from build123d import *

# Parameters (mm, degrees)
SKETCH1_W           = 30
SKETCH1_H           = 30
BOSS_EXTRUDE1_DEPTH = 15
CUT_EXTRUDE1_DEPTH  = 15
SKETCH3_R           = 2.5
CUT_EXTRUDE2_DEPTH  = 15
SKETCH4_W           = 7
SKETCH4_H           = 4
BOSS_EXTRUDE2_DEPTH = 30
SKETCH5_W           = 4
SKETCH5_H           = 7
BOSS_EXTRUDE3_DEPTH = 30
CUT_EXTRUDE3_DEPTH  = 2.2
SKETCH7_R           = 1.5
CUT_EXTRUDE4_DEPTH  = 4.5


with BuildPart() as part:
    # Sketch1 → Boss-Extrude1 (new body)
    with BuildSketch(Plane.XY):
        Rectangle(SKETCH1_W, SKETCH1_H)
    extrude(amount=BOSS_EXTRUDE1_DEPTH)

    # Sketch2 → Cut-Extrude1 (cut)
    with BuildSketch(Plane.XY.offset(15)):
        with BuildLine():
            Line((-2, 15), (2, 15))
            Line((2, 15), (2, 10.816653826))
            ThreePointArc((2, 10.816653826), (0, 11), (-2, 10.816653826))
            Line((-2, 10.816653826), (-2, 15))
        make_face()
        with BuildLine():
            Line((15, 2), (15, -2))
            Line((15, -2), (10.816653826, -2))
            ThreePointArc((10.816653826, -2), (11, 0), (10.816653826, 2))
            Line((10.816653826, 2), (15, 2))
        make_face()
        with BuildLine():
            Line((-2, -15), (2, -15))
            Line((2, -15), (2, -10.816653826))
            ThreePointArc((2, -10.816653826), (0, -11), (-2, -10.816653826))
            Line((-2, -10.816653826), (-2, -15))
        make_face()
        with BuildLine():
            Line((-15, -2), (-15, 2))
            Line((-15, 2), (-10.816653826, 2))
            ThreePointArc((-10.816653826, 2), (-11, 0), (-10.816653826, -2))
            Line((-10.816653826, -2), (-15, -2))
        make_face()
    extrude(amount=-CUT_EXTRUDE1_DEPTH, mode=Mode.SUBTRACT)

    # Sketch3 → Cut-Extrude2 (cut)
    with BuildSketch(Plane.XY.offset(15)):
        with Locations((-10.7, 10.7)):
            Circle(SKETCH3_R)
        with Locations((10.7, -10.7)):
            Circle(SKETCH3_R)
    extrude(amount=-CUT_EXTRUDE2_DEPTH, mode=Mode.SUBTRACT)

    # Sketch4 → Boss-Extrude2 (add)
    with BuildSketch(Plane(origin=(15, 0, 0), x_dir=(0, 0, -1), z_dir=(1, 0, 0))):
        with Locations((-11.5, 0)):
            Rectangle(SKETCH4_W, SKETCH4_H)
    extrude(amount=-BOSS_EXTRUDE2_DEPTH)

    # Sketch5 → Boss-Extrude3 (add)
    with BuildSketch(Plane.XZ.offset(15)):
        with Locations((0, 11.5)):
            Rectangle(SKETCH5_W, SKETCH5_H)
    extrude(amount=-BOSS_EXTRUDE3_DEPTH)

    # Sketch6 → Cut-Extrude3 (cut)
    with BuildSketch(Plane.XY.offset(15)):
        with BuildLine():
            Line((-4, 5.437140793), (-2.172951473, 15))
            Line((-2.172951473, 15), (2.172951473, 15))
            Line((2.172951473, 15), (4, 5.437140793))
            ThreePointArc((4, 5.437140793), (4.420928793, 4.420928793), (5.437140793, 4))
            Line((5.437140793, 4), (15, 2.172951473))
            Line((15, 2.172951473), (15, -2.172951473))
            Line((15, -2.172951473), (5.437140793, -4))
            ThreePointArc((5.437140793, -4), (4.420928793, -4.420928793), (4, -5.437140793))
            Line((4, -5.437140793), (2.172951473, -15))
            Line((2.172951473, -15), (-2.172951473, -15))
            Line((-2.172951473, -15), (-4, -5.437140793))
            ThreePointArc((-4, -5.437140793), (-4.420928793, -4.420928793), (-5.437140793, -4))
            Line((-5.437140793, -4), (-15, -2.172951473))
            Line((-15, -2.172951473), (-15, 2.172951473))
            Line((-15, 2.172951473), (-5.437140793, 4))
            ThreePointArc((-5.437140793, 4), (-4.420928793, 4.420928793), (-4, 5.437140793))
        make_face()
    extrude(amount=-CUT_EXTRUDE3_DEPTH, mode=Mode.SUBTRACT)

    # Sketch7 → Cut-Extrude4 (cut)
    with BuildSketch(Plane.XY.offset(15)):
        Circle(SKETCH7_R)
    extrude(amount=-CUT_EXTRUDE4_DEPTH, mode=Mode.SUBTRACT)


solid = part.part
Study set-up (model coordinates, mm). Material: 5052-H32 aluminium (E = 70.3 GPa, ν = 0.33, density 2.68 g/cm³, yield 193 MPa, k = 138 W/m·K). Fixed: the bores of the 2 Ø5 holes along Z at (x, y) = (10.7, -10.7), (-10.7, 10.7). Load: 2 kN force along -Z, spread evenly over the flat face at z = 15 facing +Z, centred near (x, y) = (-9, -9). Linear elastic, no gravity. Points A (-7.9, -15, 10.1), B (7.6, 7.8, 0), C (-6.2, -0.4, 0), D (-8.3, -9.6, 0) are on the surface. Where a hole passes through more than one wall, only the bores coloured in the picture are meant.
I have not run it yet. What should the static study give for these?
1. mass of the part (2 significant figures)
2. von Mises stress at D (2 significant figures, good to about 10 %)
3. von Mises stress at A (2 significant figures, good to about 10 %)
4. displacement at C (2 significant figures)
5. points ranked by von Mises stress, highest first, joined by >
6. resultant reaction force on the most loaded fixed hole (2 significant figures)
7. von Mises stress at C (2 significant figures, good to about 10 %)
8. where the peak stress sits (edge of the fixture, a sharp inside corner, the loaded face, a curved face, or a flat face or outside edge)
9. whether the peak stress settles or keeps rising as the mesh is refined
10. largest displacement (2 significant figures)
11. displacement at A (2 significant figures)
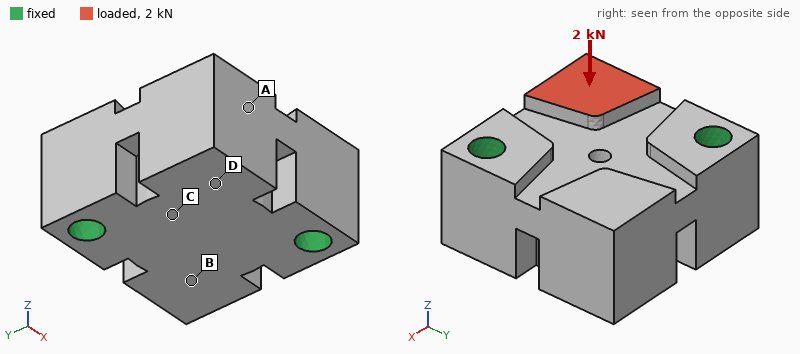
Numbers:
31 g
11 MPa
20 MPa
7.9 µm
C > A > D > B
1.0 kN
26 MPa
edge of the fixture
keeps rising
29 µm
20 µm
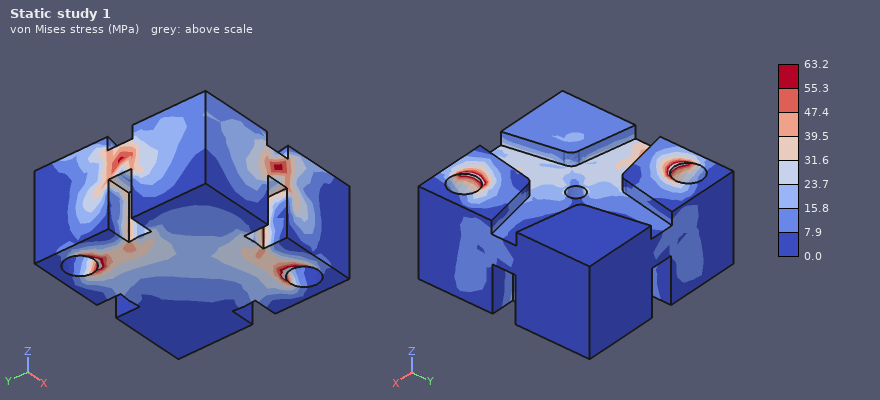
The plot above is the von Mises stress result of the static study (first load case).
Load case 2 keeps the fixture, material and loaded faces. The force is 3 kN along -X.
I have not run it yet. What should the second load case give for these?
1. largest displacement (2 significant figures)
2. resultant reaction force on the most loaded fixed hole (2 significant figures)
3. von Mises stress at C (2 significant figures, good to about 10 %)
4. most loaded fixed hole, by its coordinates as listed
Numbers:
30 µm
2.5 kN
26 MPa
(10.7, -10.7)
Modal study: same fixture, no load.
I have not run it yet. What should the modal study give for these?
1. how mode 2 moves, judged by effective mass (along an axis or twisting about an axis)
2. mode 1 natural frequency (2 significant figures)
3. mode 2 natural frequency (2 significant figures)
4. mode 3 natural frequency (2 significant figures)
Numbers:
along Z
19 kHz
24 kHz
35 kHz
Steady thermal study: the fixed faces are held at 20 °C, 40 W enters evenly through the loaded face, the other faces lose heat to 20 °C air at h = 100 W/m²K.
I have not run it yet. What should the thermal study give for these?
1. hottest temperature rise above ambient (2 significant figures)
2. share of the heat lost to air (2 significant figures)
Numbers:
29 K
5.0 %
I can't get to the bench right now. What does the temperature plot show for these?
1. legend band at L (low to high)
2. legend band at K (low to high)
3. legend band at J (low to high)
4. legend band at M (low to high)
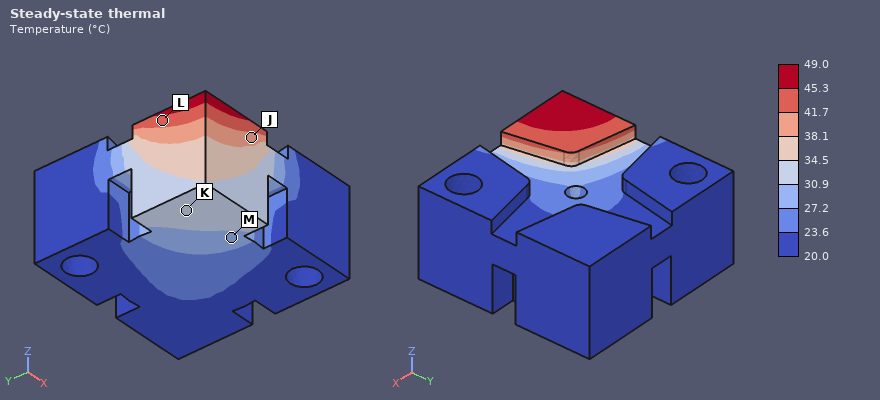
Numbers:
41.7 to 45.3 °C
30.9 to 34.5 °C
38.1 to 41.7 °C
27.2 to 30.9 °C
